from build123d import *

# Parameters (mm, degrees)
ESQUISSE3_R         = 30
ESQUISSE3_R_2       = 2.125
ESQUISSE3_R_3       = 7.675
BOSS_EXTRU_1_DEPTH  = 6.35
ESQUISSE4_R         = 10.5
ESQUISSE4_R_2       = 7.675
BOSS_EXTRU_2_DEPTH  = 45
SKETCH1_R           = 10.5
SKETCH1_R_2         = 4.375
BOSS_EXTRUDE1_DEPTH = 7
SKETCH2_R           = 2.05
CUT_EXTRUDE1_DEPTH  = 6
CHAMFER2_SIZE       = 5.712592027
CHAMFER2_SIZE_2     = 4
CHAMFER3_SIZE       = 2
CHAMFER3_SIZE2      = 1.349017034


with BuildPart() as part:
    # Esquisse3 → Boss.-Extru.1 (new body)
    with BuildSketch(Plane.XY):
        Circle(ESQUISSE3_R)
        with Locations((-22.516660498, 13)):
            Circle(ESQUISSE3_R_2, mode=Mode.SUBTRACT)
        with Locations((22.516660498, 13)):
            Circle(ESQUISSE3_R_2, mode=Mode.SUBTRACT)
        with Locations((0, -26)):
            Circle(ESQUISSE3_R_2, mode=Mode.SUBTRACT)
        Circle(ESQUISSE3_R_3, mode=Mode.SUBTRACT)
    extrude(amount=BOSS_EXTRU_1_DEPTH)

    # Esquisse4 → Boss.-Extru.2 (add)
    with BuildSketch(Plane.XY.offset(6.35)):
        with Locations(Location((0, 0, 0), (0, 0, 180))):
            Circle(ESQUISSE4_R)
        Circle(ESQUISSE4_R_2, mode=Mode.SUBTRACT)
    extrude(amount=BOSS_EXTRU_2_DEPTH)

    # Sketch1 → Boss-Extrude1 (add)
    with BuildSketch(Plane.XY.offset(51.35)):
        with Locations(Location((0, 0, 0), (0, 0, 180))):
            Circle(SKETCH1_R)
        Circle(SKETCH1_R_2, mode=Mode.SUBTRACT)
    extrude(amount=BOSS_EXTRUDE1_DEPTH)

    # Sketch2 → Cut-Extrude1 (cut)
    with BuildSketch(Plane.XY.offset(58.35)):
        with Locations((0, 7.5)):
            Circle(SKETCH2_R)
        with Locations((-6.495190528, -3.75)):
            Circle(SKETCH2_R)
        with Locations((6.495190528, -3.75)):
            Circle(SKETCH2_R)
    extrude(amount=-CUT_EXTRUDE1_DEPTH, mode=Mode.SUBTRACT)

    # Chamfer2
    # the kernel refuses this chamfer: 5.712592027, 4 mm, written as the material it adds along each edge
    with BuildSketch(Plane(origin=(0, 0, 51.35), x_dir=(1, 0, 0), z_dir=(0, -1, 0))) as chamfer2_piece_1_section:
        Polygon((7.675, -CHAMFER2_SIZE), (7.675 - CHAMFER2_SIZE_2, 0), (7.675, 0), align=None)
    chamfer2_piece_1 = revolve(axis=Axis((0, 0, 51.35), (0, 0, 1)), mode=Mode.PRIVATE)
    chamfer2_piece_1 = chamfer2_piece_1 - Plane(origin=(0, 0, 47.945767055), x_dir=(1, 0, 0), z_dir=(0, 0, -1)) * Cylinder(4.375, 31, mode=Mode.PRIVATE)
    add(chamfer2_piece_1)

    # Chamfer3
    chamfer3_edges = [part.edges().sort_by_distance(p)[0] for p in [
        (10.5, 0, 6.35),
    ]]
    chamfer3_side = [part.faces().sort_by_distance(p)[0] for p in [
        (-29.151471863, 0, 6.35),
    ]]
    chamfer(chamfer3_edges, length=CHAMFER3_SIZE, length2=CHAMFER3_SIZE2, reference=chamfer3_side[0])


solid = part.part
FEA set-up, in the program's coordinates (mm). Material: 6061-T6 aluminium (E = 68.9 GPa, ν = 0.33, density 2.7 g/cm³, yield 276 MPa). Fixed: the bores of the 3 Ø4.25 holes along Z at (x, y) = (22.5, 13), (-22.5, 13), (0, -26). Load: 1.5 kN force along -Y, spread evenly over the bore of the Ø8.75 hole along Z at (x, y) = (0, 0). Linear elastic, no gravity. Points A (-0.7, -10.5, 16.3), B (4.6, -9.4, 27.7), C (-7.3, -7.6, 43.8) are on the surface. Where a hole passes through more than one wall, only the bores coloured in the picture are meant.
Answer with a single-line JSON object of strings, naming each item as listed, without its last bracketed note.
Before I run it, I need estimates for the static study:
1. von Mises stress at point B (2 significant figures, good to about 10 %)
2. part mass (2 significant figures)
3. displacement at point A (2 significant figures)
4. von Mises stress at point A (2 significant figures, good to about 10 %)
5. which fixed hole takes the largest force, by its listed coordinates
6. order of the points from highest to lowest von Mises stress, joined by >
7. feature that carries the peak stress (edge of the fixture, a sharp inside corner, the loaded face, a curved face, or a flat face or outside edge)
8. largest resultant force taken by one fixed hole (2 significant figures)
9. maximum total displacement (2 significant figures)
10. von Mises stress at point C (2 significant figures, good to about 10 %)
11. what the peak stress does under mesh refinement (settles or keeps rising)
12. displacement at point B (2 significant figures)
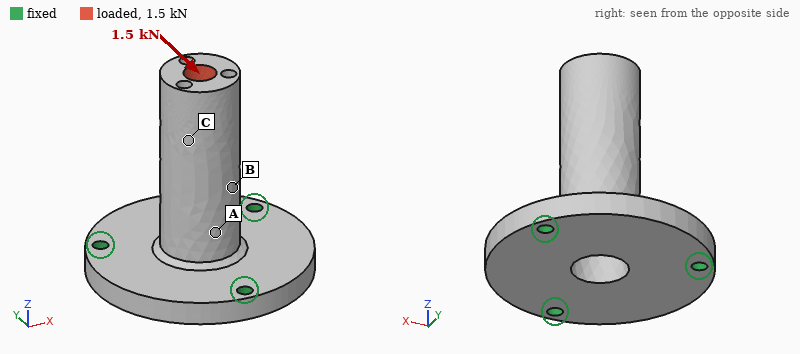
{"von Mises stress at point B": "56 MPa", "part mass": "70 g", "displacement at point A": "0.070 mm", "von Mises stress at point A": "82 MPa", "which fixed hole takes the largest force, by its listed coordinates": "(0, -26)", "order of the points from highest to lowest von Mises stress, joined by >": "A > B > C", "feature that carries the peak stress": "edge of the fixture", "largest resultant force taken by one fixed hole": "2.2 kN", "maximum total displacement": "0.34 mm", "von Mises stress at point C": "23 MPa", "what the peak stress does under mesh refinement": "keeps rising", "displacement at point B": "0.13 mm"}
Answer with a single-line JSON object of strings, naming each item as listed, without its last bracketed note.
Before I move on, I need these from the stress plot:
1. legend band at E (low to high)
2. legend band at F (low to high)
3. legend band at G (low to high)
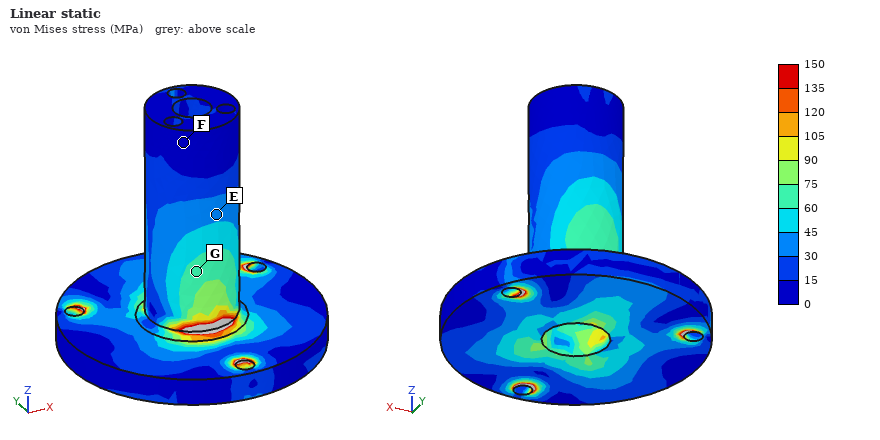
{"legend band at E": "30 to 45 MPa", "legend band at F": "0 to 15 MPa", "legend band at G": "60 to 75 MPa"}
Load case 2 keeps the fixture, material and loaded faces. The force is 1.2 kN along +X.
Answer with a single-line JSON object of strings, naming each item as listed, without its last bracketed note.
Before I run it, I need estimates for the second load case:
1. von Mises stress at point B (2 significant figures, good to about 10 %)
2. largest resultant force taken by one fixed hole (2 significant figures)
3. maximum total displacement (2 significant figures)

{"von Mises stress at point B": "31 MPa", "largest resultant force taken by one fixed hole": "1.5 kN", "maximum total displacement": "0.27 mm"}
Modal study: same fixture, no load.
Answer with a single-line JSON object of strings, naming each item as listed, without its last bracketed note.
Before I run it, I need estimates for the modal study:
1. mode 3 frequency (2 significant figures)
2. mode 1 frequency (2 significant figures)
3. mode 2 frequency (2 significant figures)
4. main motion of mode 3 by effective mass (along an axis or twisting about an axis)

{"mode 3 frequency": "8600 Hz", "mode 1 frequency": "3300 Hz", "mode 2 frequency": "3300 Hz", "main motion of mode 3 by effective mass": "along Z"}
